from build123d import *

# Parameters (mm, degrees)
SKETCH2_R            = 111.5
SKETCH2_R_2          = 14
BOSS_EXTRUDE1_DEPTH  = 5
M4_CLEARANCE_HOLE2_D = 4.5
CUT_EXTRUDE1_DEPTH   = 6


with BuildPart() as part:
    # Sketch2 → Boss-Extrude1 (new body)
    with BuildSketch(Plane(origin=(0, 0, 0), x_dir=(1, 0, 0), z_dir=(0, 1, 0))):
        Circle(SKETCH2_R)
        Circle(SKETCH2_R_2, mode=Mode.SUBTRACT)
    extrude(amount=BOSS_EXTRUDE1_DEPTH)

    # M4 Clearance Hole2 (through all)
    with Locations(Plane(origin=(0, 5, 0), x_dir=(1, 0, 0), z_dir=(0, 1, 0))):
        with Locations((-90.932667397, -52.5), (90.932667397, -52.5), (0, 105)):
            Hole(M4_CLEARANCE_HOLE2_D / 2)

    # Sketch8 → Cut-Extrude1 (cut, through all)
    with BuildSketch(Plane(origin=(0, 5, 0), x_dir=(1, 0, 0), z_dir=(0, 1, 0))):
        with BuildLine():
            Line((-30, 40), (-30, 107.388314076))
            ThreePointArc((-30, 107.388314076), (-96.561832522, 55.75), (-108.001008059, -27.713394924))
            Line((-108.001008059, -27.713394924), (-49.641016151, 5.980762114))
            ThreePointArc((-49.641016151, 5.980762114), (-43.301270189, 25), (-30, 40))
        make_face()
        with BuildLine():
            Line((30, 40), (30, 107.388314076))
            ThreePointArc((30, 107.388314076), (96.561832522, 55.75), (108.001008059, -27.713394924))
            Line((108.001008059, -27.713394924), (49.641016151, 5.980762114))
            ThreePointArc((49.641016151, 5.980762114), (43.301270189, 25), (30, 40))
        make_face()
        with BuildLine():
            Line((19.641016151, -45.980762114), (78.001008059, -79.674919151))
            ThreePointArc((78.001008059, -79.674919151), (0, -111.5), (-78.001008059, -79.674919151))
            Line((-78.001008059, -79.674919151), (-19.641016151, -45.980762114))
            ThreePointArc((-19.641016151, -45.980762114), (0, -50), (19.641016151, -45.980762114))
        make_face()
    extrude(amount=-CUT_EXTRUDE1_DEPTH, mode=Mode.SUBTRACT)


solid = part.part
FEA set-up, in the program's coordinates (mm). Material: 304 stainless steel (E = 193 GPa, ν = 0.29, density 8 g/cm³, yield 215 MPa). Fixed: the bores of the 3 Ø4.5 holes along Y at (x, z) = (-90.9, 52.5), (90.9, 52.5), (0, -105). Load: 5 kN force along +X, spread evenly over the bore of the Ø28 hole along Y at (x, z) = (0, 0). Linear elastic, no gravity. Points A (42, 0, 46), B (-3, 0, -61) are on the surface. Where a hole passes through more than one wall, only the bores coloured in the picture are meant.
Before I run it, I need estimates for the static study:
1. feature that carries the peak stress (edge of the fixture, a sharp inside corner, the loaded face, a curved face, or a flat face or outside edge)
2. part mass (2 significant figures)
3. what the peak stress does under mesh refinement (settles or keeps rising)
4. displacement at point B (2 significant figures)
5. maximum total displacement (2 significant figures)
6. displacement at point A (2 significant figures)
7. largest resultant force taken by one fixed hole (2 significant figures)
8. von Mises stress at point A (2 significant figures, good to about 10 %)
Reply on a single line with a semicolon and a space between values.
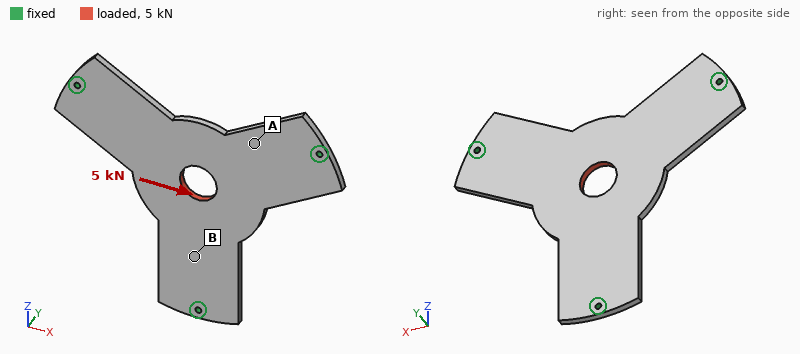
edge of the fixture; 740 g; keeps rising; 5.7 µm; 11 µm; 4.2 µm; 2.6 kN; 10 MPa
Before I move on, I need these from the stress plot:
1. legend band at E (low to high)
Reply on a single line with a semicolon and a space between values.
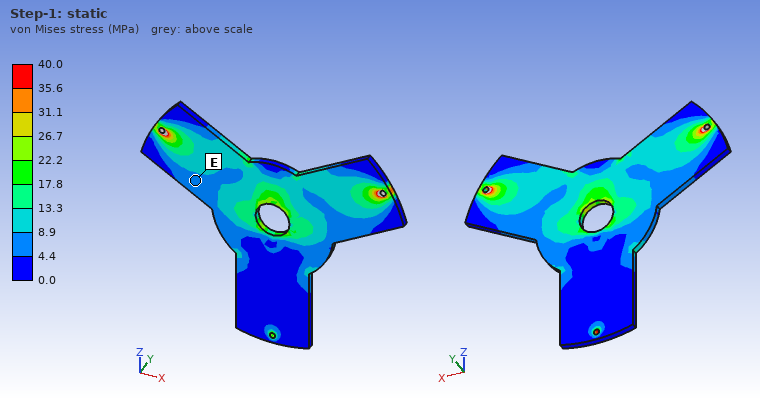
4.4 to 8.9 MPa
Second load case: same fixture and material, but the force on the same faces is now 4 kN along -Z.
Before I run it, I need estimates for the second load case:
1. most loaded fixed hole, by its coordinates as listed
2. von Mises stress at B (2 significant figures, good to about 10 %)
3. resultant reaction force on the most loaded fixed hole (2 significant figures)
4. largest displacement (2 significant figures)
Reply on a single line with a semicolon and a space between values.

(0, -105); 8.8 MPa; 2.4 kN; 8.7 µm
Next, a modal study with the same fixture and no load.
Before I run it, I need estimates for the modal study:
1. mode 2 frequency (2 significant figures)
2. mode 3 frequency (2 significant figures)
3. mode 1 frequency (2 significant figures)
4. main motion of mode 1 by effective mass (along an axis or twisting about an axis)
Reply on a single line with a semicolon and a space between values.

1200 Hz; 1200 Hz; 600 Hz; along Y
